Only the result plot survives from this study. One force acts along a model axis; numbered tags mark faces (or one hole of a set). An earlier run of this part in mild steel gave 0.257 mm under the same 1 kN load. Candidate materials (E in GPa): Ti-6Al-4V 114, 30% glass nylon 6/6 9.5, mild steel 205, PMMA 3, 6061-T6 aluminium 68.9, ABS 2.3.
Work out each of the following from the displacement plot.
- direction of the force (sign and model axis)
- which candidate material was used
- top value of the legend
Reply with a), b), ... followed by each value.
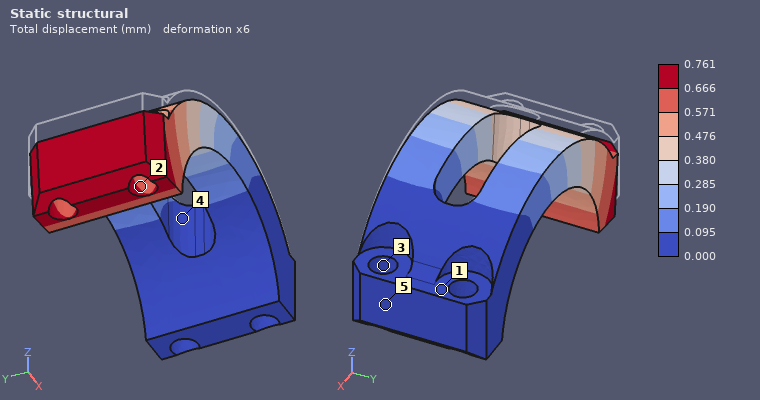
a) -Z
b) 6061-T6 aluminium
c) 0.761 mm
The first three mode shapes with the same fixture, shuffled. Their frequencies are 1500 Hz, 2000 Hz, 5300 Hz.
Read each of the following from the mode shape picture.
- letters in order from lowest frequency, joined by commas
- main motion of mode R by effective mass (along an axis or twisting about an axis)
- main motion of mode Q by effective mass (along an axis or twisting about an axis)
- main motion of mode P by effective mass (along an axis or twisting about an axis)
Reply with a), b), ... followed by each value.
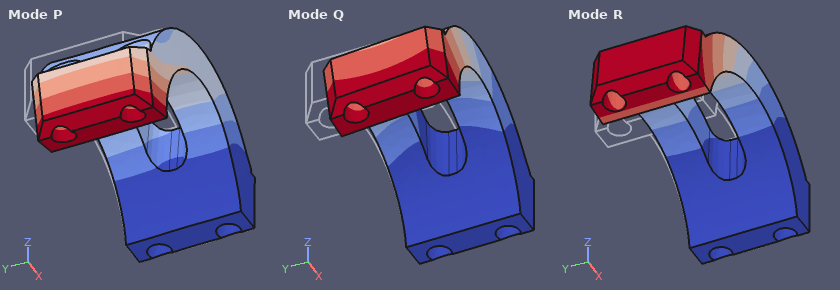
a) R, Q, P
b) along Z
c) along Y
d) along X
